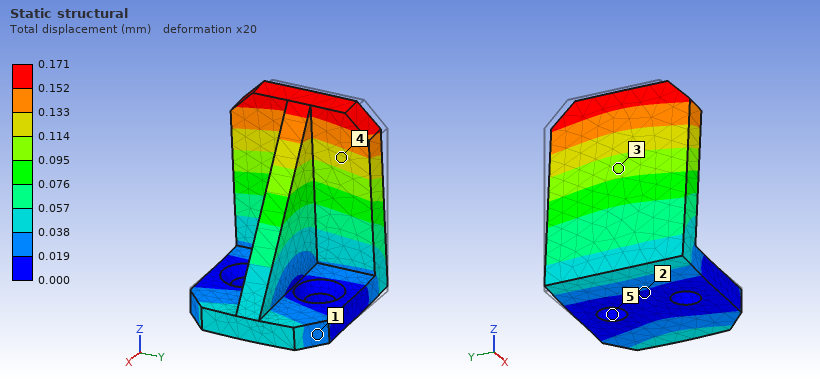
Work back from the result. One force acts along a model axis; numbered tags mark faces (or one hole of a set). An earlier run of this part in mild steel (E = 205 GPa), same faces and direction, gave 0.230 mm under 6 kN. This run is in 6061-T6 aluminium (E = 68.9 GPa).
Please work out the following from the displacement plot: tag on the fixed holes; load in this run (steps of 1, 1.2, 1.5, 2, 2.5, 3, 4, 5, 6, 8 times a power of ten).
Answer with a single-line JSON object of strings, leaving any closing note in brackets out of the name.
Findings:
{"tag on the fixed holes": "5", "load in this run": "1.5 kN"}
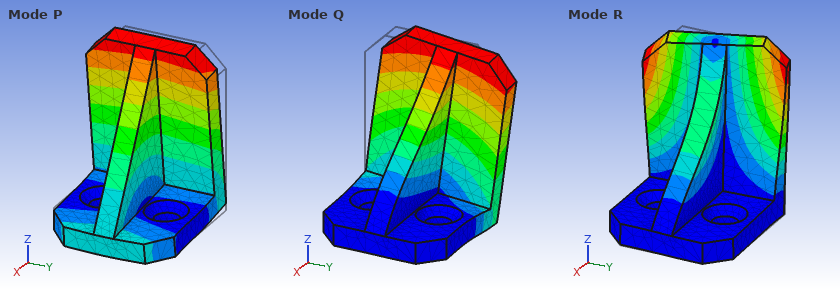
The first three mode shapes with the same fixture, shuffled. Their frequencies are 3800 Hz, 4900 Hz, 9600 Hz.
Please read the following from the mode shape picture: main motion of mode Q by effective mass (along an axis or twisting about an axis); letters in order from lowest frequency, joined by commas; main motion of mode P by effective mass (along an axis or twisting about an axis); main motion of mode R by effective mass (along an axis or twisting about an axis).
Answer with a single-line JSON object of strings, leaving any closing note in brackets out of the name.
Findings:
{"main motion of mode Q by effective mass": "along Y", "letters in order from lowest frequency, joined by commas": "P, Q, R", "main motion of mode P by effective mass": "along X", "main motion of mode R by effective mass": "twisting about Z"}
